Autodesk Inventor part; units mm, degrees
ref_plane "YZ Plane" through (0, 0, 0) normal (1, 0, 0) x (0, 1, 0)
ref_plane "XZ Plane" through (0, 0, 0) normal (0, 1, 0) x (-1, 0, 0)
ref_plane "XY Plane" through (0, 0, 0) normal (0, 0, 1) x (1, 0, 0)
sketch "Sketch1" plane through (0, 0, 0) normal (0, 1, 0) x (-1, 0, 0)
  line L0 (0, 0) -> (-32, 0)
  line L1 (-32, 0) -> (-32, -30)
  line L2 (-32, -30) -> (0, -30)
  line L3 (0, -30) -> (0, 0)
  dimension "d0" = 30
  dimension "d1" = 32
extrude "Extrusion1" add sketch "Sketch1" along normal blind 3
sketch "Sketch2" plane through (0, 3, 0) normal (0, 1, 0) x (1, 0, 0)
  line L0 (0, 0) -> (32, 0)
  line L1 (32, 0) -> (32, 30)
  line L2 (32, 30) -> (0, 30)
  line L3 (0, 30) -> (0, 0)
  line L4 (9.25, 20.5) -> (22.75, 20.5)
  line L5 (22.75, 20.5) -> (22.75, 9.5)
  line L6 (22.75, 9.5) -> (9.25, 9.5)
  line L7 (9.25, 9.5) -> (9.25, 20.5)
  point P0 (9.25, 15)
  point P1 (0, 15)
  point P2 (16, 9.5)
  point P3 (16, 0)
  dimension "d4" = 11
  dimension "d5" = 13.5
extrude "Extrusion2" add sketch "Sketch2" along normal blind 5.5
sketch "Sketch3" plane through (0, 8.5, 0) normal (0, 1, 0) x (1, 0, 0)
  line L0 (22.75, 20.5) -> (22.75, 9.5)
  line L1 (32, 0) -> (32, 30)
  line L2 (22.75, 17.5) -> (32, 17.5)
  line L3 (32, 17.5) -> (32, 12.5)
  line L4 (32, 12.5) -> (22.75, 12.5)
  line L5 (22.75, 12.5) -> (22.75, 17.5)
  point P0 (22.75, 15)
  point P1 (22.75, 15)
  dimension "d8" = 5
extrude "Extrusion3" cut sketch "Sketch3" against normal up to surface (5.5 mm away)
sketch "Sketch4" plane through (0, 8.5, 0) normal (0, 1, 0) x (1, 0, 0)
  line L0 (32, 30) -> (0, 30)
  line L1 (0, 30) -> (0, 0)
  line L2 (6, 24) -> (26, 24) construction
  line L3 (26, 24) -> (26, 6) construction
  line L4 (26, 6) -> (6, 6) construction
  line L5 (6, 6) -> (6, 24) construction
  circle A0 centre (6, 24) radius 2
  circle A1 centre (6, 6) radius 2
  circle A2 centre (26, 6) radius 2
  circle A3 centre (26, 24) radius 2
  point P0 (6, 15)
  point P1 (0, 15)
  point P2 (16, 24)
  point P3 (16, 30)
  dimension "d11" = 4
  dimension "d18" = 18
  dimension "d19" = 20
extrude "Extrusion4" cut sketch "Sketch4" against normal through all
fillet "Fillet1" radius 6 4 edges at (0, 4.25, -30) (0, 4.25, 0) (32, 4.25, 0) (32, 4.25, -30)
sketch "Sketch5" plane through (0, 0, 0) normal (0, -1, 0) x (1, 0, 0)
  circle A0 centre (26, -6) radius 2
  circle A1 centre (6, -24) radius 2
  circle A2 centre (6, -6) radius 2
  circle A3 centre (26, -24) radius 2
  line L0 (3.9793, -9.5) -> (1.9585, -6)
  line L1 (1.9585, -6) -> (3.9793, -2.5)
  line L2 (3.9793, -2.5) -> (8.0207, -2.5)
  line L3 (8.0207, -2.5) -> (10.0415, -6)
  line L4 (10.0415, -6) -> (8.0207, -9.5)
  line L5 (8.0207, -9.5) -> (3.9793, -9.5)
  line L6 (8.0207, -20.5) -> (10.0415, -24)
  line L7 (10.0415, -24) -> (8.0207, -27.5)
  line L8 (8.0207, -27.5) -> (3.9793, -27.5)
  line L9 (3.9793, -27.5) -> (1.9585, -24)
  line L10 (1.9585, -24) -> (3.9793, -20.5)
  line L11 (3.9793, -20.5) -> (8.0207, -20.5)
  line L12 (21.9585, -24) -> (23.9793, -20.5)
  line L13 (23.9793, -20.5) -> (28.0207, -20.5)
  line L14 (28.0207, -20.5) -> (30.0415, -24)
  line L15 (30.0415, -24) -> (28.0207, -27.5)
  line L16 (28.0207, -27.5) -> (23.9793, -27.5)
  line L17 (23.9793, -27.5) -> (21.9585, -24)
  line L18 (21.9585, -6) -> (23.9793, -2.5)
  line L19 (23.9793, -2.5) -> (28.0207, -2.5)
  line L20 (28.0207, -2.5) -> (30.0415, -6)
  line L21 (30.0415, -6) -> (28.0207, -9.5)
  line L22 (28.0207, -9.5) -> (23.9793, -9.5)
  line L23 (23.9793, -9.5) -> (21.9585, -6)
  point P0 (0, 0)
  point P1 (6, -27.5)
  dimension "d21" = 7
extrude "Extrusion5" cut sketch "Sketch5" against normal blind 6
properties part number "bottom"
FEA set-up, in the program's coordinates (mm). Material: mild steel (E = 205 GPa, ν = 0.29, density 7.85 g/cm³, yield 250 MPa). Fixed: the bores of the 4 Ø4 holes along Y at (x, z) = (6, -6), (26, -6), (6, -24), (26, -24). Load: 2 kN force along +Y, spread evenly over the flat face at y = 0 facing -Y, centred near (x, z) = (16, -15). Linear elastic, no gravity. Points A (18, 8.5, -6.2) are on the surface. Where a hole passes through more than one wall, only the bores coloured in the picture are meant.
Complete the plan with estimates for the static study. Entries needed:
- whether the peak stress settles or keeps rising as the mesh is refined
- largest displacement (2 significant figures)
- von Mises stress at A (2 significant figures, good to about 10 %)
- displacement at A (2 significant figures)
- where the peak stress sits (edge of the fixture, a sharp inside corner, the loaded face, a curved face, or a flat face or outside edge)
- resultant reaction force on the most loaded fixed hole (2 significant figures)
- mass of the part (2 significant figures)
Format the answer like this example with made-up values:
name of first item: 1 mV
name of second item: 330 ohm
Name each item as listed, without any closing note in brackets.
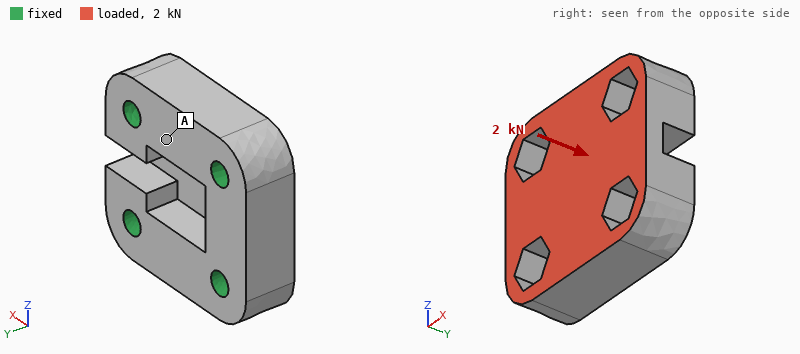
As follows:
whether the peak stress settles or keeps rising as the mesh is refined: keeps rising
largest displacement: 1.5 µm
von Mises stress at A: 6.2 MPa
displacement at A: 0.88 µm
where the peak stress sits: edge of the fixture
resultant reaction force on the most loaded fixed hole: 530 N
mass of the part: 45 g
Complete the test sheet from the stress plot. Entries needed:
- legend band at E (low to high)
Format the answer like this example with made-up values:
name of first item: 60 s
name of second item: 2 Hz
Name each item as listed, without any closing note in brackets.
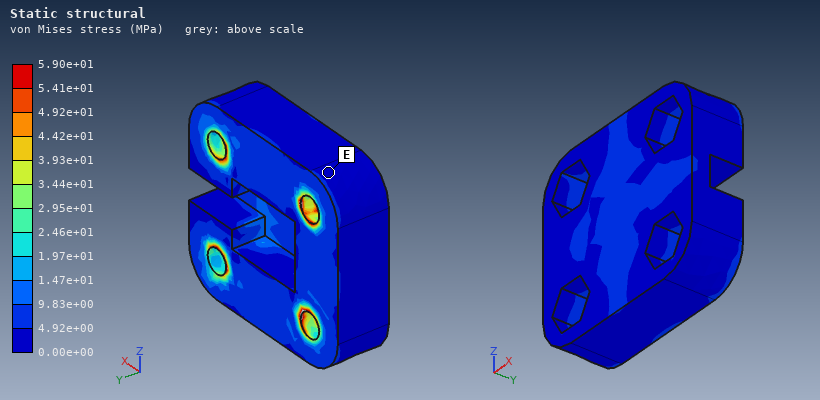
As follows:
legend band at E: 0.00e+00 to 4.92e+00 MPa
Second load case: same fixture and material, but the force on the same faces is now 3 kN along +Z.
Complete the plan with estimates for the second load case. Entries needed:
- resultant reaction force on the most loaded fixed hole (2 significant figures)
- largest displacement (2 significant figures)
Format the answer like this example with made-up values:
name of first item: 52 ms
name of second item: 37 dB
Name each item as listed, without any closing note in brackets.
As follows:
resultant reaction force on the most loaded fixed hole: 1.0 kN
largest displacement: 4.0 µm
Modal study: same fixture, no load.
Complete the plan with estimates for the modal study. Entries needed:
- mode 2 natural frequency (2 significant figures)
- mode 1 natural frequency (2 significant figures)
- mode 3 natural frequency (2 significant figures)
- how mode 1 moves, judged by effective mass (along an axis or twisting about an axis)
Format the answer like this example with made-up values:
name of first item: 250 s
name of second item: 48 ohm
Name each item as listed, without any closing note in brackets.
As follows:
mode 2 natural frequency: 38 kHz
mode 1 natural frequency: 33 kHz
mode 3 natural frequency: 39 kHz
how mode 1 moves, judged by effective mass: along Z
